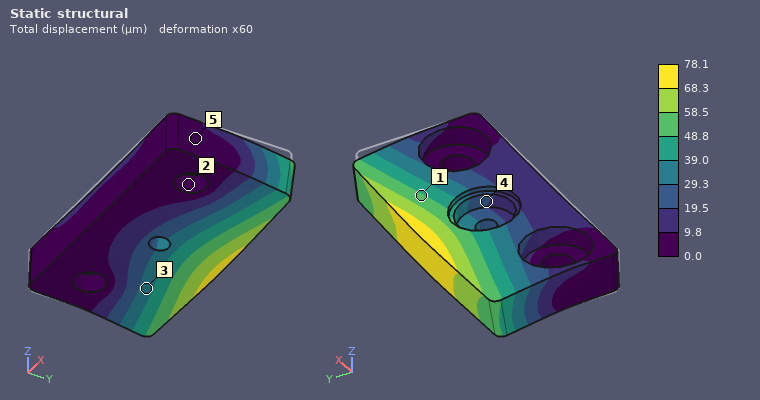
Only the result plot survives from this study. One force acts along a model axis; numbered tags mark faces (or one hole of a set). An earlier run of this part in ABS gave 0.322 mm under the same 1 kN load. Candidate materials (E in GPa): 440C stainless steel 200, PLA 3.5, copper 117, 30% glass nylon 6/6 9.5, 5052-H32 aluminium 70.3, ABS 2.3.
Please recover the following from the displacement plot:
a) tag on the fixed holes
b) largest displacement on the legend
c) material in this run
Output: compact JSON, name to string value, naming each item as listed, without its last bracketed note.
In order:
{"tag on the fixed holes": "2", "largest displacement on the legend": "78.1 µm", "material in this run": "30% glass nylon 6/6"}
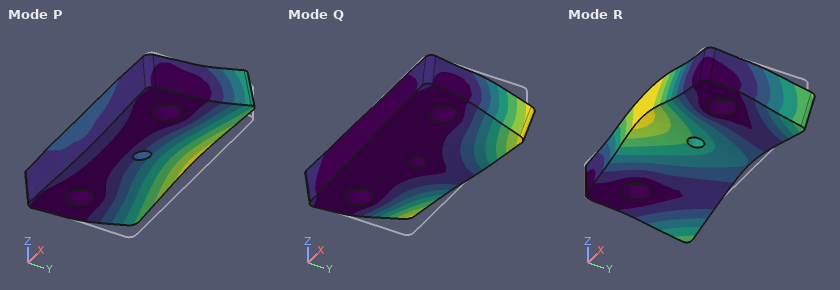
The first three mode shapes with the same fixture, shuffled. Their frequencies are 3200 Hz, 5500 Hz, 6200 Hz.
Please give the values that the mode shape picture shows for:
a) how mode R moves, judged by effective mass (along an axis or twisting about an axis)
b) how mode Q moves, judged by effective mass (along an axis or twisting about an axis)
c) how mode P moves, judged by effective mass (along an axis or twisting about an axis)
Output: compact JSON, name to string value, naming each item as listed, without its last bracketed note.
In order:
{"how mode R moves, judged by effective mass": "along Z", "how mode Q moves, judged by effective mass": "twisting about Y", "how mode P moves, judged by effective mass": "along Z"}
